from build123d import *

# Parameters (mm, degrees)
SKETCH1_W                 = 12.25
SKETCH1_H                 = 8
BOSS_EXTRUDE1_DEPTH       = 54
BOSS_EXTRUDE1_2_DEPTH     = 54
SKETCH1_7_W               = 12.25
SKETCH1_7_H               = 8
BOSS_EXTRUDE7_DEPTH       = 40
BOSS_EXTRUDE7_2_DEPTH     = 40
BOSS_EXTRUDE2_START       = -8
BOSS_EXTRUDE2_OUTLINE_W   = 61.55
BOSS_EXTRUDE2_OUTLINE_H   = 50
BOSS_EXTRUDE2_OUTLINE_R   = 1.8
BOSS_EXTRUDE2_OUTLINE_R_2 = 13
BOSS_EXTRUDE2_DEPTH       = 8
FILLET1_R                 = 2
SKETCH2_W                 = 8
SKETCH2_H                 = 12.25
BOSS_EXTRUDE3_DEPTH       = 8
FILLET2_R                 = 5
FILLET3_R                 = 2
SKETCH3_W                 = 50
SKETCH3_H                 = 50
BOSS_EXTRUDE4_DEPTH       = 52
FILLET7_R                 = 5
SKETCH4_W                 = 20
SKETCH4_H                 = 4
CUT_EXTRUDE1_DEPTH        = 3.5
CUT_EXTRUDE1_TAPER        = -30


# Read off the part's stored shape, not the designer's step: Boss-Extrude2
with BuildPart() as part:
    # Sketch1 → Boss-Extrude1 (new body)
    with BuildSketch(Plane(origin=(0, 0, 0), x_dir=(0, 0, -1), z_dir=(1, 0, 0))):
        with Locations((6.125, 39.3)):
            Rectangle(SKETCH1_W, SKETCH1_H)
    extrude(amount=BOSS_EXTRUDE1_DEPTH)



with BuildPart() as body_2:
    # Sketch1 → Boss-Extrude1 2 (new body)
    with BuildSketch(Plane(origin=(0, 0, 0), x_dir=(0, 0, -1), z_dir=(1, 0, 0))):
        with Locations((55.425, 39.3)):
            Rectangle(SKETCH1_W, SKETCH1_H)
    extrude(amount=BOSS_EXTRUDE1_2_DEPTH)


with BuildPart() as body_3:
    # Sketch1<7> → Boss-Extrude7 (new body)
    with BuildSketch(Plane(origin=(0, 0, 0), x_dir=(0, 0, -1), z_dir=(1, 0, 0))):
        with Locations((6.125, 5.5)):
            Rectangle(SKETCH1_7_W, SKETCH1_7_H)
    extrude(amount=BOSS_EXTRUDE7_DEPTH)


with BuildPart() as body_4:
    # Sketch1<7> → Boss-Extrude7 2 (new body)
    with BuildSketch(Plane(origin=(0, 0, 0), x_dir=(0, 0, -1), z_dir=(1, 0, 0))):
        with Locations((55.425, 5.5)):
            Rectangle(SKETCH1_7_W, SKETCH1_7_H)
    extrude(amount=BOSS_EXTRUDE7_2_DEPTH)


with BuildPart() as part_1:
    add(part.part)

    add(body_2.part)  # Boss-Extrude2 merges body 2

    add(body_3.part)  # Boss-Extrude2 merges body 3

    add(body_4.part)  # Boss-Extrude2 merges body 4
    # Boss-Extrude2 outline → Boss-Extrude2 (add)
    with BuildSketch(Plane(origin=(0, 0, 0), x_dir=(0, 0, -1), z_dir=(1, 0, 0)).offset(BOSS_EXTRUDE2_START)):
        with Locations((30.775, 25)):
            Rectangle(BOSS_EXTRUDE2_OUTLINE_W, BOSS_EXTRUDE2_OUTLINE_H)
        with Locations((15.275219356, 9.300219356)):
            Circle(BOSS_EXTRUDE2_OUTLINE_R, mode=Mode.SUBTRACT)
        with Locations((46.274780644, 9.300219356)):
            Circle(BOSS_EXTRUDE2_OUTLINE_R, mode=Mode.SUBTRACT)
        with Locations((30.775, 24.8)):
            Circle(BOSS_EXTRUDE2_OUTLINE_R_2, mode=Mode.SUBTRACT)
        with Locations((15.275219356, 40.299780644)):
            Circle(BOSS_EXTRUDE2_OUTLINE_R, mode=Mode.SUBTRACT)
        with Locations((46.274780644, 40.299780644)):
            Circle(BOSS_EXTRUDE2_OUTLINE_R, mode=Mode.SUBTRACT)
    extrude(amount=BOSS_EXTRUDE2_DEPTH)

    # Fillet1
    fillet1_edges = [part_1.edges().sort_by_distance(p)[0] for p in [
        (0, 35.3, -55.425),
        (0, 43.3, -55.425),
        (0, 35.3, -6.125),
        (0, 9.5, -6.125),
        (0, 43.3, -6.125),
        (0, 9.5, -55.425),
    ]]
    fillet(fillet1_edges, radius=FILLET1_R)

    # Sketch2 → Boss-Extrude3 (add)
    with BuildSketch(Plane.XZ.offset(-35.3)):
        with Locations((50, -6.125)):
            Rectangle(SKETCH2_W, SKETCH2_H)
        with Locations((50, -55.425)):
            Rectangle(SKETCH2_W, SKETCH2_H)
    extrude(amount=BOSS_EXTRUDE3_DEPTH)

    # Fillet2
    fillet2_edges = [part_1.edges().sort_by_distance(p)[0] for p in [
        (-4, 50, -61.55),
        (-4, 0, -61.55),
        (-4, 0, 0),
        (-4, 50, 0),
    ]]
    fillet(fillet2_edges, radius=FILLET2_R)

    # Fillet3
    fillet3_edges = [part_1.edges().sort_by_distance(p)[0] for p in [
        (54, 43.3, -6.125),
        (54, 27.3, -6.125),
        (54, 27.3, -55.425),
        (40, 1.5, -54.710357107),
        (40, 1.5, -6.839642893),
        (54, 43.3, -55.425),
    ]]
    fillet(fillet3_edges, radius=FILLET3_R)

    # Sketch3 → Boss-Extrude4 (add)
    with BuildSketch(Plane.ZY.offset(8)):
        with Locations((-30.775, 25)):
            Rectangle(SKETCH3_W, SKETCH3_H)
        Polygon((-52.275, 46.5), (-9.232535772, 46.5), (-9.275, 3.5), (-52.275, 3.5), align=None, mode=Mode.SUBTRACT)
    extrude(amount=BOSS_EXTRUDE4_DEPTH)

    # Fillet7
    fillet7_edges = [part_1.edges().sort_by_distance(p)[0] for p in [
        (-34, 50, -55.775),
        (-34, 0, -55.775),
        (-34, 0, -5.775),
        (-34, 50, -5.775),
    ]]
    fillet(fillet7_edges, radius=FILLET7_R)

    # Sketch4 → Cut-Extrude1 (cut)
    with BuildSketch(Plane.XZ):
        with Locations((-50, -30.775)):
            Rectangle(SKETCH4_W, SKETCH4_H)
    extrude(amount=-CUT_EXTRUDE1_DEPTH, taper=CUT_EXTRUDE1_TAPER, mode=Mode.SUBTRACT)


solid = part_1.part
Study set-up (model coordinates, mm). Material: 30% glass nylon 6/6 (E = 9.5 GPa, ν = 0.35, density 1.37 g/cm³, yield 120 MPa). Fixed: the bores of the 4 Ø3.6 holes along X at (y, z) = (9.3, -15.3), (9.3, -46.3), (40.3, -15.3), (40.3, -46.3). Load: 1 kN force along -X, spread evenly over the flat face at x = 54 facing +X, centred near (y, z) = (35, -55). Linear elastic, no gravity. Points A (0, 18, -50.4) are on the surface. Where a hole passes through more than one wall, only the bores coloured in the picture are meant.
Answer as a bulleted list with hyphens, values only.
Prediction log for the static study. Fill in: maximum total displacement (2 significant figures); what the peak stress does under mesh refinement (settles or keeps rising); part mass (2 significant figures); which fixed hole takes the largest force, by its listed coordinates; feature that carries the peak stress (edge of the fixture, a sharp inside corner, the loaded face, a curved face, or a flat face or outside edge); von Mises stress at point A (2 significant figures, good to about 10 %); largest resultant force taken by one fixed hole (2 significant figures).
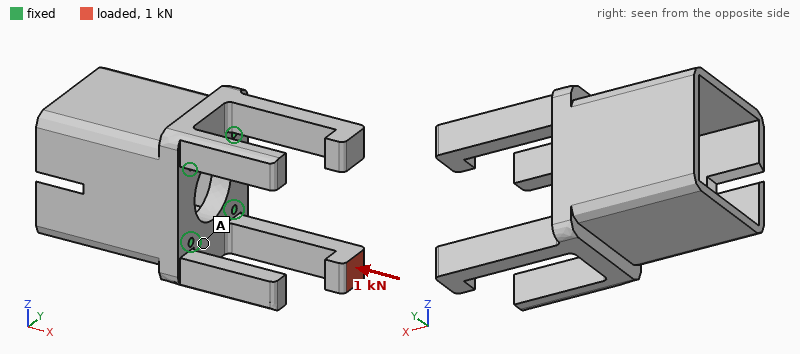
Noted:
- 1.4 mm
- keeps rising
- 99 g
- (40.3, -46.3)
- edge of the fixture
- 4.7 MPa
- 900 N
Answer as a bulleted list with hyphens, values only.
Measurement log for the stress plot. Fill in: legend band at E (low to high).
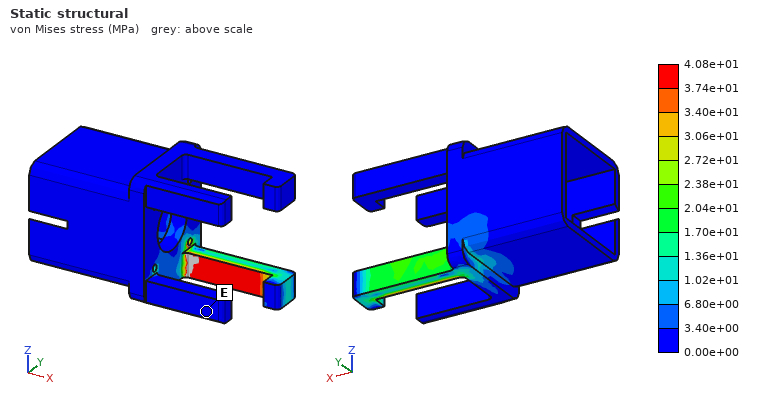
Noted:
- 0.00e+00 to 3.40e+00 MPa
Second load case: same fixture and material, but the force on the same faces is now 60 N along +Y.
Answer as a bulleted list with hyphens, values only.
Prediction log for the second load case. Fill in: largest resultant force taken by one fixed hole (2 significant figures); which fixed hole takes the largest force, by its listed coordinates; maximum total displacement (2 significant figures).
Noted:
- 96 N
- (40.3, -46.3)
- 0.76 mm
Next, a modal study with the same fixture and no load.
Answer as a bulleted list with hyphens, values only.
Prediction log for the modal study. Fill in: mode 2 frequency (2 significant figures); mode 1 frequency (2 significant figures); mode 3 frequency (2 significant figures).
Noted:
- 870 Hz
- 870 Hz
- 1100 Hz
